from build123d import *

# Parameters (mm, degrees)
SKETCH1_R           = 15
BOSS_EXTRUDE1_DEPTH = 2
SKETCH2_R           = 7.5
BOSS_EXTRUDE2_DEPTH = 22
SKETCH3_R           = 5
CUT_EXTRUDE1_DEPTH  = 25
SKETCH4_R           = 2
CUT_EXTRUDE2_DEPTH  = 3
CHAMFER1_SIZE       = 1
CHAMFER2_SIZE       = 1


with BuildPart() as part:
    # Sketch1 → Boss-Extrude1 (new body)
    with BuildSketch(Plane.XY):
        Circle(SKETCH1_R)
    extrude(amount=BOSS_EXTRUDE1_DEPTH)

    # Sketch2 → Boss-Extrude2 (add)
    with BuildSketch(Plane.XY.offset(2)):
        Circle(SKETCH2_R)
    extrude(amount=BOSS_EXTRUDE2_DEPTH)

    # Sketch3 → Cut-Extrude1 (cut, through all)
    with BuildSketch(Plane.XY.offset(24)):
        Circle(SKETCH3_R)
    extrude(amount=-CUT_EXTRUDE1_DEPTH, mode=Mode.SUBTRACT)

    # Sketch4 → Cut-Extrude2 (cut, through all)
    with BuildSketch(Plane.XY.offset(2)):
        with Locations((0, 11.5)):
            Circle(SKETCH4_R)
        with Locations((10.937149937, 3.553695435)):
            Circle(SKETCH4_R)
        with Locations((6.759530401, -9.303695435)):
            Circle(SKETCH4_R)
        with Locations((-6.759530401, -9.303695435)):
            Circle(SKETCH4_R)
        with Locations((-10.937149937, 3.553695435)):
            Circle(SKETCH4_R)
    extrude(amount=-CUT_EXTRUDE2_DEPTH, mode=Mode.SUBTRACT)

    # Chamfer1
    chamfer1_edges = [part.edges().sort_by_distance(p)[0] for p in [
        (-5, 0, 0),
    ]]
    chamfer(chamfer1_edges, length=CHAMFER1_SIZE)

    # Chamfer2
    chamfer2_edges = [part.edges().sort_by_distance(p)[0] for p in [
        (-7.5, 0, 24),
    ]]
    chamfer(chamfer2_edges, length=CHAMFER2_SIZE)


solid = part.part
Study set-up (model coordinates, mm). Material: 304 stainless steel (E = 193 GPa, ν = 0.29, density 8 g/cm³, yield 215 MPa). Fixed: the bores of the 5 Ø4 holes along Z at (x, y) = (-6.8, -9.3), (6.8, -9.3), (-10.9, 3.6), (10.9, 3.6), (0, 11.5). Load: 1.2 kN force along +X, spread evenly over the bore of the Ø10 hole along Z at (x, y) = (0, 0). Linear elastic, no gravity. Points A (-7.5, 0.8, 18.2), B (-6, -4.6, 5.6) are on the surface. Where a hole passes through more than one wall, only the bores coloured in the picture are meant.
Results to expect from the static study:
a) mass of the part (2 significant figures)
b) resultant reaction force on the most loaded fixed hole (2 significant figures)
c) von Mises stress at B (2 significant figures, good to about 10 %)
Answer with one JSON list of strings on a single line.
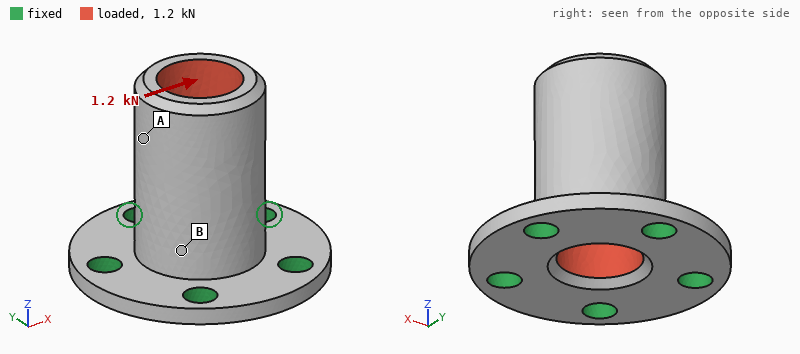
["26 g", "680 N", "29 MPa"]
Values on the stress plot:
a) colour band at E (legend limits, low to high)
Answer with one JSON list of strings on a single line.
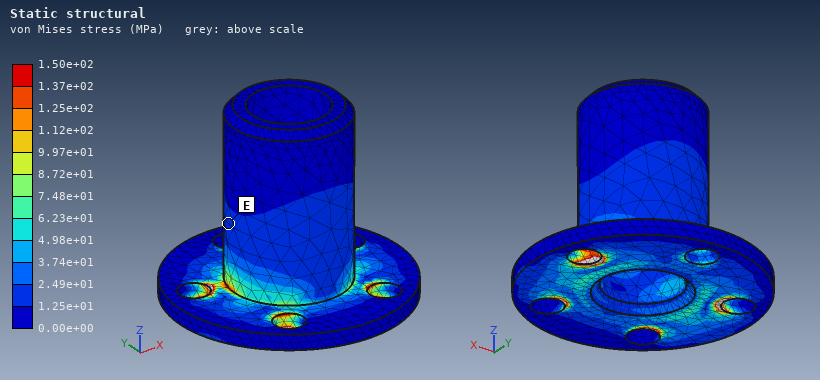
["1.25e+01 to 2.49e+01 MPa"]
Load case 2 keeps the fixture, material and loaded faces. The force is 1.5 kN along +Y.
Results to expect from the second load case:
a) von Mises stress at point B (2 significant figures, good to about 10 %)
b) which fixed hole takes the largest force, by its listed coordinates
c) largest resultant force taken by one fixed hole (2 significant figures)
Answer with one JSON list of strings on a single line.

["34 MPa", "(0, 11.5)", "890 N"]
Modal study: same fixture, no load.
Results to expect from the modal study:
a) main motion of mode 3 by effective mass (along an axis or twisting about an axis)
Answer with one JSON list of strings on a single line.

["along Z"]
